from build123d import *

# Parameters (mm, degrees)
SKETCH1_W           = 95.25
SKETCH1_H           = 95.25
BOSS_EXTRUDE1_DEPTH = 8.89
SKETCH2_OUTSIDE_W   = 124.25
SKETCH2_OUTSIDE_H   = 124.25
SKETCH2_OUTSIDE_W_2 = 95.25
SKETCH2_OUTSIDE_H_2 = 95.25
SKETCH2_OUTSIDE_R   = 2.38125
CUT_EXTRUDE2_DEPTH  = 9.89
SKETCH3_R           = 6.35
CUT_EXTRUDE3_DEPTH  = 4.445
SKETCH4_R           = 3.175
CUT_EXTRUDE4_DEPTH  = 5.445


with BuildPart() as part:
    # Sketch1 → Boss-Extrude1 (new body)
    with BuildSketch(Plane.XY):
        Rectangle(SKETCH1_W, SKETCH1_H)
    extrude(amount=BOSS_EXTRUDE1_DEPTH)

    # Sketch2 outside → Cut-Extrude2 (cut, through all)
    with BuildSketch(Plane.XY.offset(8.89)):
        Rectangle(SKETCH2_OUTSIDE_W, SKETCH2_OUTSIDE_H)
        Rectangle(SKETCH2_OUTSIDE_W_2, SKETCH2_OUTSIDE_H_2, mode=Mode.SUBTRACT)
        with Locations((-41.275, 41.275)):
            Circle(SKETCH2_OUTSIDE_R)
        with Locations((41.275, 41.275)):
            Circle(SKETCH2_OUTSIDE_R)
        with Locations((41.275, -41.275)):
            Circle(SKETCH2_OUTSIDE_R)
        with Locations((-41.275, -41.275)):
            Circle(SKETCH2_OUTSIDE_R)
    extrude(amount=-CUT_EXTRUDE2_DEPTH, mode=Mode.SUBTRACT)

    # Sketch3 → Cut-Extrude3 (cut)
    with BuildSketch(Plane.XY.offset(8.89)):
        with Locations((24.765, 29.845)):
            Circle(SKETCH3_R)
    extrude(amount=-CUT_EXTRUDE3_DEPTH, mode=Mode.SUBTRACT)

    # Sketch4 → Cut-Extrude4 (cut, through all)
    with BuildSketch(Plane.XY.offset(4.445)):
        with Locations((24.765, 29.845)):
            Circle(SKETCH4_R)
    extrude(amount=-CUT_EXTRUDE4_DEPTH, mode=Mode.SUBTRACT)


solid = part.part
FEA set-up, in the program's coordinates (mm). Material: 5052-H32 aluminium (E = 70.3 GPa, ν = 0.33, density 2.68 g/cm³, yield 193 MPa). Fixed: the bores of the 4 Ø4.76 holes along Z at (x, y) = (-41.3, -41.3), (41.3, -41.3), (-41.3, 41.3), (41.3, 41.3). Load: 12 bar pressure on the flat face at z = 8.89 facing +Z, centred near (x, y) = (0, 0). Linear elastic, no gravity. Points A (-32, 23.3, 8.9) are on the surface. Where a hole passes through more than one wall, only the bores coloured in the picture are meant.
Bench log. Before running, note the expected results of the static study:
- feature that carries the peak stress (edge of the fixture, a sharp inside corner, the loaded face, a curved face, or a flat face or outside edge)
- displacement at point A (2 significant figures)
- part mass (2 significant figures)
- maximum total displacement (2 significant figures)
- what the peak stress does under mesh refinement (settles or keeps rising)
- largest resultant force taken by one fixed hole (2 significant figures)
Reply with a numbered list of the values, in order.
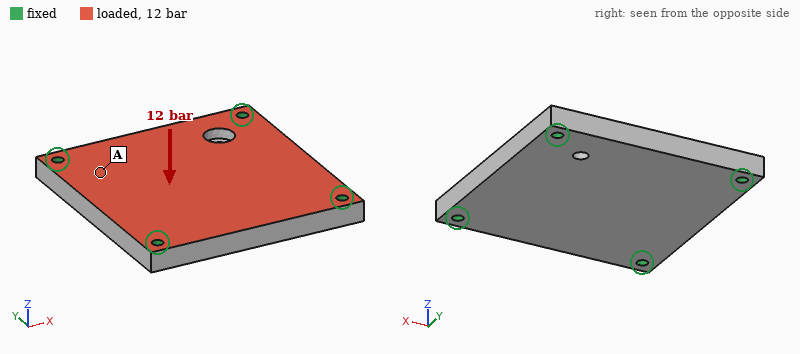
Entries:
1. edge of the fixture
2. 0.053 mm
3. 210 g
4. 0.11 mm
5. keeps rising
6. 2.7 kN
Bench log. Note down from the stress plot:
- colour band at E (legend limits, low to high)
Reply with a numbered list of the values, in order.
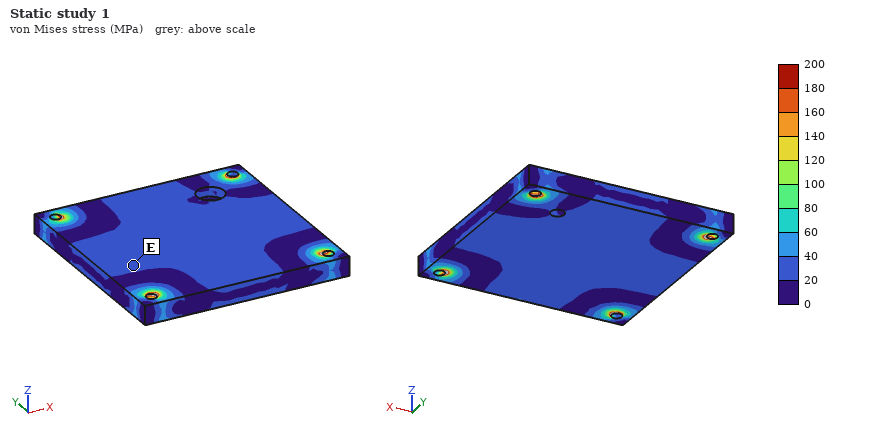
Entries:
1. 20 to 40 MPa
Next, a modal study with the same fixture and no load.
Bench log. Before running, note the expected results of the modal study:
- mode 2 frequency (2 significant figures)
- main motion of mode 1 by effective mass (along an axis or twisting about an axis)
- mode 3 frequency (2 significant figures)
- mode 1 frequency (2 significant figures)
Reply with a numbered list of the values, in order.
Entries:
1. 6800 Hz
2. along Z
3. 6800 Hz
4. 4000 Hz
